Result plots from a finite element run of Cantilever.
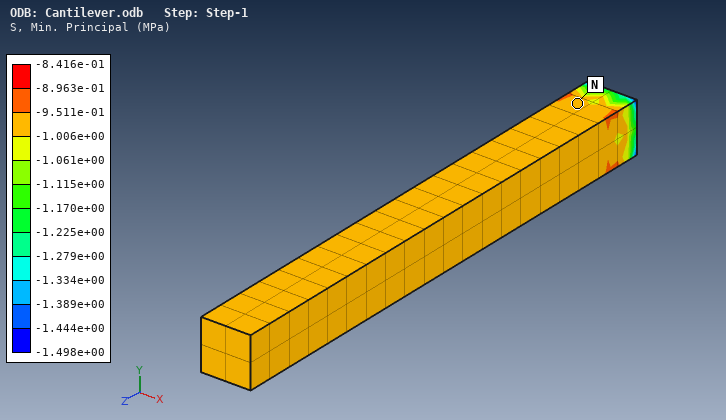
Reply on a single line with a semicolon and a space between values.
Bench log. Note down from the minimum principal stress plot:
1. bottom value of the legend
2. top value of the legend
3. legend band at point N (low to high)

-1.498e+00 MPa; -8.416e-01 MPa; -1.006e+00 to -9.511e-01 MPa
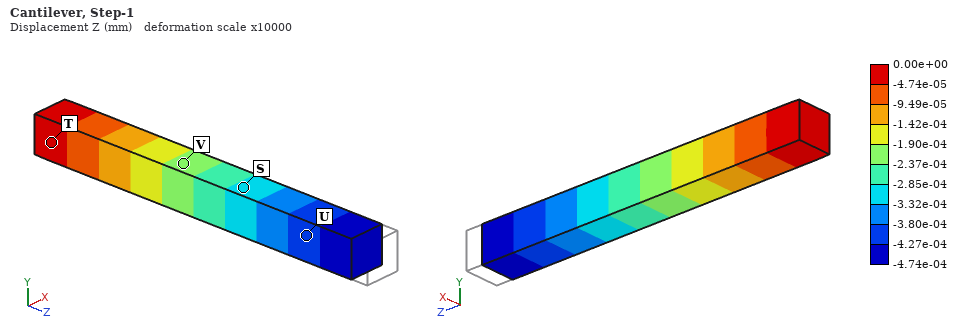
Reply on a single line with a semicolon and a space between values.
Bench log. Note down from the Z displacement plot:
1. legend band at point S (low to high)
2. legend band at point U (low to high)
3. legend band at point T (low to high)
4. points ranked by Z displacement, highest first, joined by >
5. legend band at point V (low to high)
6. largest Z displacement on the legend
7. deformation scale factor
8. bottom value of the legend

-3.32e-04 to -2.85e-04 mm; -4.27e-04 to -3.80e-04 mm; -4.74e-05 to 0.00e+00 mm; T > V > S > U; -2.37e-04 to -1.90e-04 mm; 0.00e+00 mm; 10000; -4.74e-04 mm
